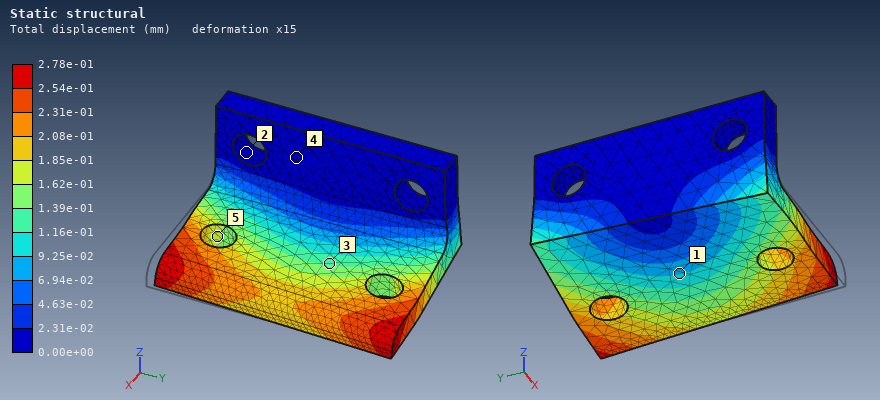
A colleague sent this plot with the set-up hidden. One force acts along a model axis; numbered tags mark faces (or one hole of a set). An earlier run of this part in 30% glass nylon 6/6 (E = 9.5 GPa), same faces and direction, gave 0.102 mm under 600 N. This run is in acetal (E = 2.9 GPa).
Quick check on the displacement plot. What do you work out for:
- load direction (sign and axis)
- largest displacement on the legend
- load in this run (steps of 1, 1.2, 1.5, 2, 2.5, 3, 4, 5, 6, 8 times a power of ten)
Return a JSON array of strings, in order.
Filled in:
["+Y", "2.78e-01 mm", "500 N"]
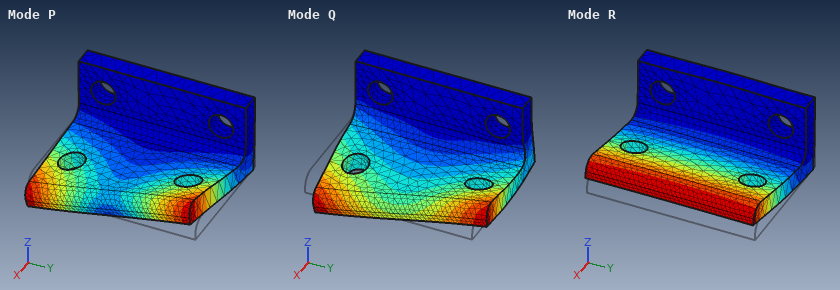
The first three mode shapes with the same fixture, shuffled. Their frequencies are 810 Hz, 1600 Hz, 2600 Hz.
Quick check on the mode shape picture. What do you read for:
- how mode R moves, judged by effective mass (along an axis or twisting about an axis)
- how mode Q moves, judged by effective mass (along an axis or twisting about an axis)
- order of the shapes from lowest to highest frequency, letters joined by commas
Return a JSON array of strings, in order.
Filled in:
["along Z", "along Y", "R, P, Q"]
